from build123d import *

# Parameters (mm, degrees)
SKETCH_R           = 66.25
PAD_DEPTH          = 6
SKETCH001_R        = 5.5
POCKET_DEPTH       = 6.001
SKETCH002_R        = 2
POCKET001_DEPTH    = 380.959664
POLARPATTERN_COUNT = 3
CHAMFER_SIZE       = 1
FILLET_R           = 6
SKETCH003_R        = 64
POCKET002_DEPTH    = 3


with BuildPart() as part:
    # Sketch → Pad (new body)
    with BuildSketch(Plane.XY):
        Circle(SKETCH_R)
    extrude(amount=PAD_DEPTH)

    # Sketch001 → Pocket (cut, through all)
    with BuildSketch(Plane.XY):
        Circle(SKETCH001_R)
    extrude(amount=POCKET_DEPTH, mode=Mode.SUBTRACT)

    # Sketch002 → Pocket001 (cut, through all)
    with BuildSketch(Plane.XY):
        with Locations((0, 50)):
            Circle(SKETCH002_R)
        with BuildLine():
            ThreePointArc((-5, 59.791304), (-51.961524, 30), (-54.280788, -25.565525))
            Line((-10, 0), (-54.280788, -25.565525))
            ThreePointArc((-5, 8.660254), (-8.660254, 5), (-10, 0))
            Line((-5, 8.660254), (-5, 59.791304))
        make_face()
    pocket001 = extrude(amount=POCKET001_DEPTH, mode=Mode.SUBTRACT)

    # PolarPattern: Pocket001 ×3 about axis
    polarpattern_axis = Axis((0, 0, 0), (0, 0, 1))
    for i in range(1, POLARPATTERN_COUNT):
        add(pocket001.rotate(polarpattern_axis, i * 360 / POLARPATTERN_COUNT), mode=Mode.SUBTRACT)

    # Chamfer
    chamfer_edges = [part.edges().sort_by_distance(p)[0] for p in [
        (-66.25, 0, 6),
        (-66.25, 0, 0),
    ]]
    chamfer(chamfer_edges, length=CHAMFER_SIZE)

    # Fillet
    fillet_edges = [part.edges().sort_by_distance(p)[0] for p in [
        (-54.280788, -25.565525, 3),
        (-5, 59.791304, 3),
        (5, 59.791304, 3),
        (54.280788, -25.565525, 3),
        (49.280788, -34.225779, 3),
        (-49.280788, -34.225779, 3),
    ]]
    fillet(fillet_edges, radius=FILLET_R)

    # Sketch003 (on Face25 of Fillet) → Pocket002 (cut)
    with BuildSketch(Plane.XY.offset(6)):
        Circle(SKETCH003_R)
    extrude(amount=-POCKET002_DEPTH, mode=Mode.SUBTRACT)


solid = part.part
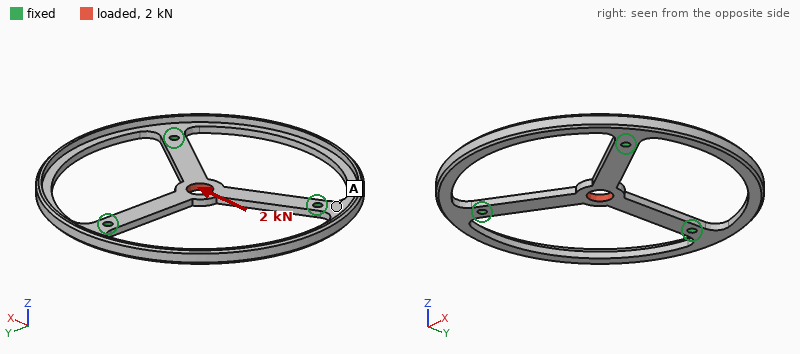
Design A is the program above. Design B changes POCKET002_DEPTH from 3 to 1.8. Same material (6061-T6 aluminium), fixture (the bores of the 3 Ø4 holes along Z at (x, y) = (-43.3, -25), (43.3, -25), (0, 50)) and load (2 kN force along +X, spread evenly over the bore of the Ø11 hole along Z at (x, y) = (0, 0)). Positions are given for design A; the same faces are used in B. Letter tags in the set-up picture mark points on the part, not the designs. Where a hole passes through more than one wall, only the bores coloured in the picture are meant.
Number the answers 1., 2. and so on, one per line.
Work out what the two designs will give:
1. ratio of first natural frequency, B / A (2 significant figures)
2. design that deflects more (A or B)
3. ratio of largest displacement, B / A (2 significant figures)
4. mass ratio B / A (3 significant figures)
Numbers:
1. 1.2
2. A
3. 0.71
4. 1.26
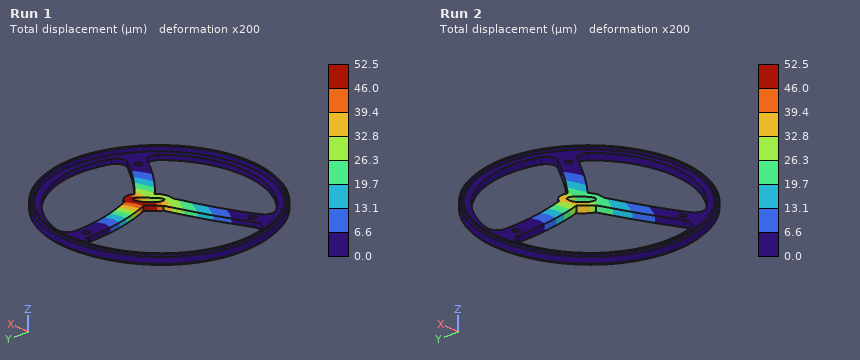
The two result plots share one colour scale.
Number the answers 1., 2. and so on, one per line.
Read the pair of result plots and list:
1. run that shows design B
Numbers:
1. Run 2
